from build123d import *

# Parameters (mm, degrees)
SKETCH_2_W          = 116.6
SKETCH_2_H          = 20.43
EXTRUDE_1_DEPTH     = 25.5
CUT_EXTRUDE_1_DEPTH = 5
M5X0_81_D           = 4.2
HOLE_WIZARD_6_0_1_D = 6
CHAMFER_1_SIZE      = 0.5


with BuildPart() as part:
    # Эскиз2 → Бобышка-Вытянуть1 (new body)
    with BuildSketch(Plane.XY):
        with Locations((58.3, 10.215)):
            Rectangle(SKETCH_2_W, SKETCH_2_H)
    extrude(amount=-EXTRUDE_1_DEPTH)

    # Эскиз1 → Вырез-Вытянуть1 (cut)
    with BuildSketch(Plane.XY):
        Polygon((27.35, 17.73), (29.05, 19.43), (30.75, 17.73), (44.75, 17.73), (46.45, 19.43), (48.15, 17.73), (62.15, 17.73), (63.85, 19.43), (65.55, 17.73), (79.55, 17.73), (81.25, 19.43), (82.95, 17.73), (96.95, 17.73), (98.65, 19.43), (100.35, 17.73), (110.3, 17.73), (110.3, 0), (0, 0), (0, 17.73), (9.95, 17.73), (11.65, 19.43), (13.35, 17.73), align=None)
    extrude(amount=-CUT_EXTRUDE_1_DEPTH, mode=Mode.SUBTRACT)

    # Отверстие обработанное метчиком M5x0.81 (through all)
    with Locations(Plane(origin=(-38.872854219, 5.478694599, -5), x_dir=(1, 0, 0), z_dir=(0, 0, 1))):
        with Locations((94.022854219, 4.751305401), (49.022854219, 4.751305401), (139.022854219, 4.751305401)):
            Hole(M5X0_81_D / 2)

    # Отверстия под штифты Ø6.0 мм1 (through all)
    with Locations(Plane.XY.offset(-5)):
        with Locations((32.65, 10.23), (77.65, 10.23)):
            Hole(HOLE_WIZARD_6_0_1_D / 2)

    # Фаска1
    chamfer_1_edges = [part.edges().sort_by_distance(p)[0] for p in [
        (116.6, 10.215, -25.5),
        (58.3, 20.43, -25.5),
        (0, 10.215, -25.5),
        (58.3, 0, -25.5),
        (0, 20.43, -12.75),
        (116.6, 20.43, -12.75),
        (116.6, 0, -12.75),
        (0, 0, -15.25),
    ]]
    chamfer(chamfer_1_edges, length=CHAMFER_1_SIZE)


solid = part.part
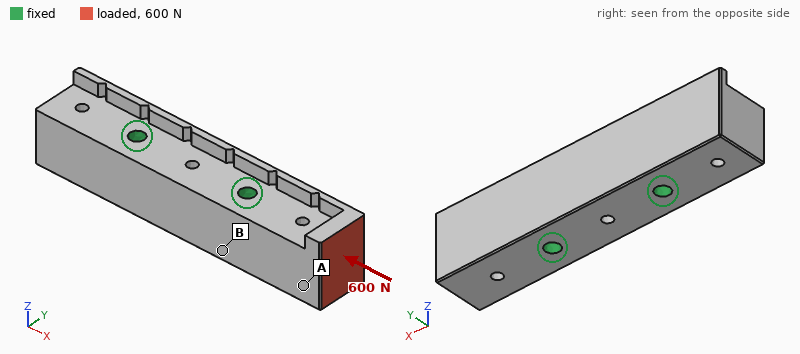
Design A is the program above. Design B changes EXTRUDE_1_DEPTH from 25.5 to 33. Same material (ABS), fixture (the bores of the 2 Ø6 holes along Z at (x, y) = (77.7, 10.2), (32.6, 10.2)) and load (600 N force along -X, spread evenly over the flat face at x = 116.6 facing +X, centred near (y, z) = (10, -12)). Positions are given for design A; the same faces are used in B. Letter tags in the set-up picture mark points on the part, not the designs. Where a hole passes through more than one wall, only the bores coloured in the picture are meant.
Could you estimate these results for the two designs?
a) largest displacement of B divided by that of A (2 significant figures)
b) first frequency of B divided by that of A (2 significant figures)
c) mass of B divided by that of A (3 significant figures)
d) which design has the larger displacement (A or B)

0.64
1.0
1.35
A
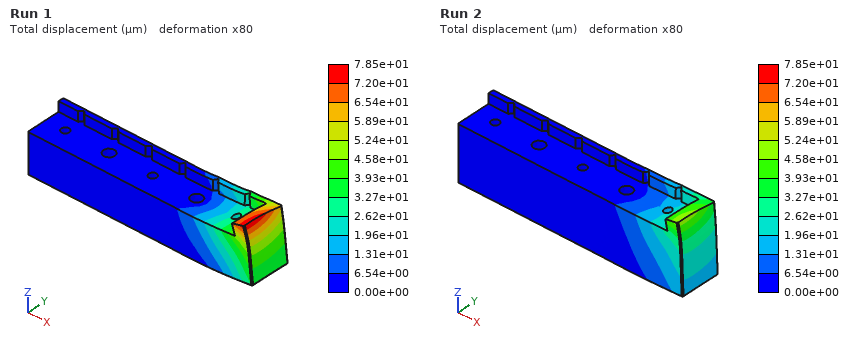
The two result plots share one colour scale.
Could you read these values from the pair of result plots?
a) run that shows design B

Run 2
